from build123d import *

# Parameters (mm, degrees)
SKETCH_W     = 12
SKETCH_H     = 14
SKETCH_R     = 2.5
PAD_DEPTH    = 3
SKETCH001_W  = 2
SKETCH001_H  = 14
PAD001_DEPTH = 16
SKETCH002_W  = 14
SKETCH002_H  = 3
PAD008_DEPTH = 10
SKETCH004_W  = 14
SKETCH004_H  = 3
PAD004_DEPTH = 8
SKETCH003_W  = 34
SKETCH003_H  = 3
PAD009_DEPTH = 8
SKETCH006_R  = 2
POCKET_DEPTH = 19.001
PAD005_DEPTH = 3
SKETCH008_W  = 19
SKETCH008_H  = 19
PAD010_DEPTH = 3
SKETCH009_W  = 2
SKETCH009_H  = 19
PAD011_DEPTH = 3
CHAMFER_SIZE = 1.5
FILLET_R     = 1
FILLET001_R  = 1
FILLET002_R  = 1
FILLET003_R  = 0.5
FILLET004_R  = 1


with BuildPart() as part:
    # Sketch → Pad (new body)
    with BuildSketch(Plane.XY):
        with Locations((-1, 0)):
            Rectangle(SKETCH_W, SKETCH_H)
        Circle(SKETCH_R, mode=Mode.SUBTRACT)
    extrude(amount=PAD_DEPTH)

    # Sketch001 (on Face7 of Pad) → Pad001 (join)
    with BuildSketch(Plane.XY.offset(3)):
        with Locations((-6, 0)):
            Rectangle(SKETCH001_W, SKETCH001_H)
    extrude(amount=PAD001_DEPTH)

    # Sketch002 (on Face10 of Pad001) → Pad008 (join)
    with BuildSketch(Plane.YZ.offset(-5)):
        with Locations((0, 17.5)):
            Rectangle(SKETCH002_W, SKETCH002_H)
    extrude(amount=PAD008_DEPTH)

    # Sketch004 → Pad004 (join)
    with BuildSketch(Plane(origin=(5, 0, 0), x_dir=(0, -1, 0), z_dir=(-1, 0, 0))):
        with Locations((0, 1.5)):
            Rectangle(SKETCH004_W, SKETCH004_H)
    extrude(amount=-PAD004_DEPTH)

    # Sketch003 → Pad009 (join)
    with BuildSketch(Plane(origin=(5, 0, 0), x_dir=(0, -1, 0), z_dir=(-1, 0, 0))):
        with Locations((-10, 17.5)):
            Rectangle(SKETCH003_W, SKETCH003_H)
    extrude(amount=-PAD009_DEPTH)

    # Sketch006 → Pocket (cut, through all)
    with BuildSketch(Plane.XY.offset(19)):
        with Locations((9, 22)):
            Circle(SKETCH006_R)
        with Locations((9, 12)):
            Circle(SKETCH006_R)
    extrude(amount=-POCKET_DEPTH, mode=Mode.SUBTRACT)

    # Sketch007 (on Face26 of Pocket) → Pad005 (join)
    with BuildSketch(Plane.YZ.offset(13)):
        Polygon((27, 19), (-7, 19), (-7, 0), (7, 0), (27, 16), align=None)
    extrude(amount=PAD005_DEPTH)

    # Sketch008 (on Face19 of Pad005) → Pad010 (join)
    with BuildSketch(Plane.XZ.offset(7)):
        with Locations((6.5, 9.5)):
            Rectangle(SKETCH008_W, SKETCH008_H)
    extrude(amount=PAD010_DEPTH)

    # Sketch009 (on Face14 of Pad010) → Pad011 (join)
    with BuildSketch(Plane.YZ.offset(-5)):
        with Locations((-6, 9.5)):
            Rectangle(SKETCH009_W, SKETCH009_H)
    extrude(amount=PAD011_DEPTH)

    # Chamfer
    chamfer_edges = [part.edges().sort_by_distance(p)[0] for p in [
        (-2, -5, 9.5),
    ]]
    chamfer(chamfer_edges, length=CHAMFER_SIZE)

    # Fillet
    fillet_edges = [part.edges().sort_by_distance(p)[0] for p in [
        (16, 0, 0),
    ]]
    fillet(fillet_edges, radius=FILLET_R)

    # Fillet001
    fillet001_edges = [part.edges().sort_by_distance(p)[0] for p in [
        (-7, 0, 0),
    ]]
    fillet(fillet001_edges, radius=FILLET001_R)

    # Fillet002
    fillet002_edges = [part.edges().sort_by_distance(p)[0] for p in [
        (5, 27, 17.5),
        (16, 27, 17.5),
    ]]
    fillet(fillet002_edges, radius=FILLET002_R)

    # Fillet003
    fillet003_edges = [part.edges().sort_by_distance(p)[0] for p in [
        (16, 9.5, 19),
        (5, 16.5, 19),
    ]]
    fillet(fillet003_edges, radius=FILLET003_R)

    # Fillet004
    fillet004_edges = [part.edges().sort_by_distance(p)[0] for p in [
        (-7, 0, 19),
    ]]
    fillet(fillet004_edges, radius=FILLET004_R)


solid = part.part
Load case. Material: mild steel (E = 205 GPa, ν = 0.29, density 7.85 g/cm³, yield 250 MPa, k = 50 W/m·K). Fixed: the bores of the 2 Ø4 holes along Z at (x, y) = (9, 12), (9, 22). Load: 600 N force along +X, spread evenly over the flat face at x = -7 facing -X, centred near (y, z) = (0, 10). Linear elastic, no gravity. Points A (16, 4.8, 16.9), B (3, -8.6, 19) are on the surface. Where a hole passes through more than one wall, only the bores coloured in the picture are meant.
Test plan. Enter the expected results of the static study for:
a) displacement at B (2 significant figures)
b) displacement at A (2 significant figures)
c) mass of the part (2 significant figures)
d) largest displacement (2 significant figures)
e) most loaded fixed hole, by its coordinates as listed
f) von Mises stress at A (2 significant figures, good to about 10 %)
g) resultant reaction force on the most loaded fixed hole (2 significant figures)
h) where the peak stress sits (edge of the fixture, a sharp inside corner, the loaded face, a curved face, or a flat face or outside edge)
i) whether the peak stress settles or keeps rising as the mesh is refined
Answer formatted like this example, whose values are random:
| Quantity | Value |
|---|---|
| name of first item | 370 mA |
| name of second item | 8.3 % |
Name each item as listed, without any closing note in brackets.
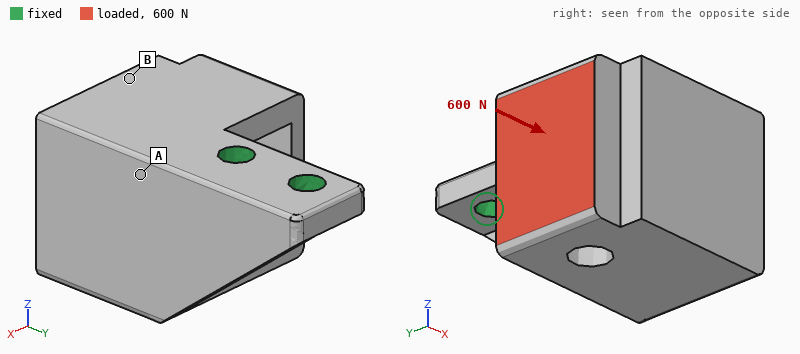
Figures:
| Quantity | Value |
|---|---|
| displacement at B | 20 µm |
| displacement at A | 15 µm |
| mass of the part | 39 g |
| largest displacement | 85 µm |
| most loaded fixed hole, by its coordinates as listed | (9, 12) |
| von Mises stress at A | 53 MPa |
| resultant reaction force on the most loaded fixed hole | 930 N |
| where the peak stress sits | edge of the fixture |
| whether the peak stress settles or keeps rising as the mesh is refined | keeps rising |
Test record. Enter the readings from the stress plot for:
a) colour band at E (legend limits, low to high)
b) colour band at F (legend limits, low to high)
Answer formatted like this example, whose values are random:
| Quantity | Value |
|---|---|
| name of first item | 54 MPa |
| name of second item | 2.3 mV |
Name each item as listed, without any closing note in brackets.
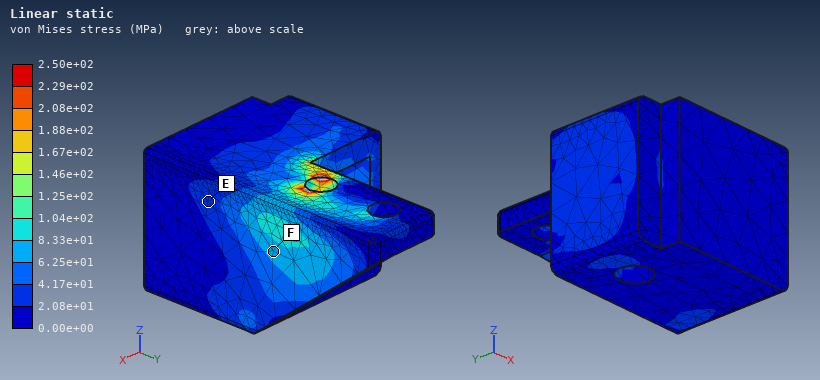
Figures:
| Quantity | Value |
|---|---|
| colour band at E | 2.08e+01 to 4.17e+01 MPa |
| colour band at F | 6.25e+01 to 8.33e+01 MPa |
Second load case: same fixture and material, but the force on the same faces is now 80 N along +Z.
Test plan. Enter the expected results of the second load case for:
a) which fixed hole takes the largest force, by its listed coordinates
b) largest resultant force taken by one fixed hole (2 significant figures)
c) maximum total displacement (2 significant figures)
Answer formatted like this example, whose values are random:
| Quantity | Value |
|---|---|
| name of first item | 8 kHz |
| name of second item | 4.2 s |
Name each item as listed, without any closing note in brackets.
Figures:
| Quantity | Value |
|---|---|
| which fixed hole takes the largest force, by its listed coordinates | (9, 12) |
| largest resultant force taken by one fixed hole | 110 N |
| maximum total displacement | 23 µm |
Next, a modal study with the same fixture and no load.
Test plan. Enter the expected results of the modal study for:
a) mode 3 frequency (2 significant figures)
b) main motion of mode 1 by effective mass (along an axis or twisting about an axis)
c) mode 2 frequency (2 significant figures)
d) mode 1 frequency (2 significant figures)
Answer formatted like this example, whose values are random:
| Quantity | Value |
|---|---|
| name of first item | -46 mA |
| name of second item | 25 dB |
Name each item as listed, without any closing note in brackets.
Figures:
| Quantity | Value |
|---|---|
| mode 3 frequency | 6800 Hz |
| main motion of mode 1 by effective mass | along X |
| mode 2 frequency | 3700 Hz |
| mode 1 frequency | 2500 Hz |
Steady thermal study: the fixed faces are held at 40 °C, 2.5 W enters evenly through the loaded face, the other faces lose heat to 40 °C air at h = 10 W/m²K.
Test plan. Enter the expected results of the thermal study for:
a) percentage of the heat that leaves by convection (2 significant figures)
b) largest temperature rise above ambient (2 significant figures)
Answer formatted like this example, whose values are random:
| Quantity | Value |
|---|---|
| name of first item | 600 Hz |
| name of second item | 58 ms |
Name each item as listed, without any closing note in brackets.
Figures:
| Quantity | Value |
|---|---|
| percentage of the heat that leaves by convection | 13 % |
| largest temperature rise above ambient | 18 K |
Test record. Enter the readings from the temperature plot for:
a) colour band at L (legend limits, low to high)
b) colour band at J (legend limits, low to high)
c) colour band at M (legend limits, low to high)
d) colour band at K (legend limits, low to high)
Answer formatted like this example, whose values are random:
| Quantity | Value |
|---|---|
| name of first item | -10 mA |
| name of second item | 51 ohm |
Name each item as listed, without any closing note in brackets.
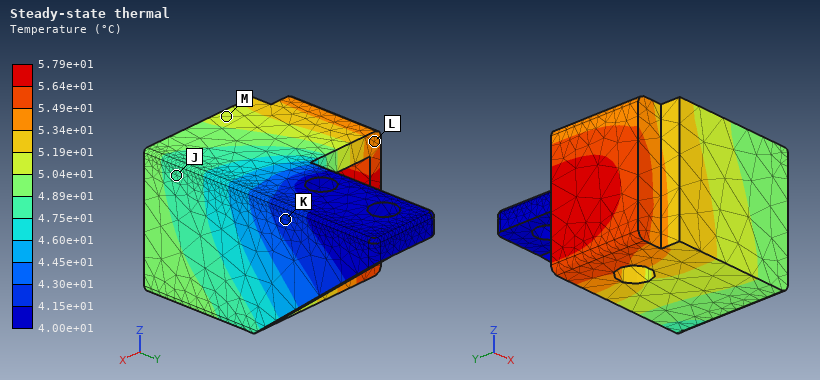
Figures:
| Quantity | Value |
|---|---|
| colour band at L | 5.34e+01 to 5.49e+01 °C |
| colour band at J | 4.75e+01 to 4.89e+01 °C |
| colour band at M | 5.04e+01 to 5.19e+01 °C |
| colour band at K | 4.15e+01 to 4.30e+01 °C |
